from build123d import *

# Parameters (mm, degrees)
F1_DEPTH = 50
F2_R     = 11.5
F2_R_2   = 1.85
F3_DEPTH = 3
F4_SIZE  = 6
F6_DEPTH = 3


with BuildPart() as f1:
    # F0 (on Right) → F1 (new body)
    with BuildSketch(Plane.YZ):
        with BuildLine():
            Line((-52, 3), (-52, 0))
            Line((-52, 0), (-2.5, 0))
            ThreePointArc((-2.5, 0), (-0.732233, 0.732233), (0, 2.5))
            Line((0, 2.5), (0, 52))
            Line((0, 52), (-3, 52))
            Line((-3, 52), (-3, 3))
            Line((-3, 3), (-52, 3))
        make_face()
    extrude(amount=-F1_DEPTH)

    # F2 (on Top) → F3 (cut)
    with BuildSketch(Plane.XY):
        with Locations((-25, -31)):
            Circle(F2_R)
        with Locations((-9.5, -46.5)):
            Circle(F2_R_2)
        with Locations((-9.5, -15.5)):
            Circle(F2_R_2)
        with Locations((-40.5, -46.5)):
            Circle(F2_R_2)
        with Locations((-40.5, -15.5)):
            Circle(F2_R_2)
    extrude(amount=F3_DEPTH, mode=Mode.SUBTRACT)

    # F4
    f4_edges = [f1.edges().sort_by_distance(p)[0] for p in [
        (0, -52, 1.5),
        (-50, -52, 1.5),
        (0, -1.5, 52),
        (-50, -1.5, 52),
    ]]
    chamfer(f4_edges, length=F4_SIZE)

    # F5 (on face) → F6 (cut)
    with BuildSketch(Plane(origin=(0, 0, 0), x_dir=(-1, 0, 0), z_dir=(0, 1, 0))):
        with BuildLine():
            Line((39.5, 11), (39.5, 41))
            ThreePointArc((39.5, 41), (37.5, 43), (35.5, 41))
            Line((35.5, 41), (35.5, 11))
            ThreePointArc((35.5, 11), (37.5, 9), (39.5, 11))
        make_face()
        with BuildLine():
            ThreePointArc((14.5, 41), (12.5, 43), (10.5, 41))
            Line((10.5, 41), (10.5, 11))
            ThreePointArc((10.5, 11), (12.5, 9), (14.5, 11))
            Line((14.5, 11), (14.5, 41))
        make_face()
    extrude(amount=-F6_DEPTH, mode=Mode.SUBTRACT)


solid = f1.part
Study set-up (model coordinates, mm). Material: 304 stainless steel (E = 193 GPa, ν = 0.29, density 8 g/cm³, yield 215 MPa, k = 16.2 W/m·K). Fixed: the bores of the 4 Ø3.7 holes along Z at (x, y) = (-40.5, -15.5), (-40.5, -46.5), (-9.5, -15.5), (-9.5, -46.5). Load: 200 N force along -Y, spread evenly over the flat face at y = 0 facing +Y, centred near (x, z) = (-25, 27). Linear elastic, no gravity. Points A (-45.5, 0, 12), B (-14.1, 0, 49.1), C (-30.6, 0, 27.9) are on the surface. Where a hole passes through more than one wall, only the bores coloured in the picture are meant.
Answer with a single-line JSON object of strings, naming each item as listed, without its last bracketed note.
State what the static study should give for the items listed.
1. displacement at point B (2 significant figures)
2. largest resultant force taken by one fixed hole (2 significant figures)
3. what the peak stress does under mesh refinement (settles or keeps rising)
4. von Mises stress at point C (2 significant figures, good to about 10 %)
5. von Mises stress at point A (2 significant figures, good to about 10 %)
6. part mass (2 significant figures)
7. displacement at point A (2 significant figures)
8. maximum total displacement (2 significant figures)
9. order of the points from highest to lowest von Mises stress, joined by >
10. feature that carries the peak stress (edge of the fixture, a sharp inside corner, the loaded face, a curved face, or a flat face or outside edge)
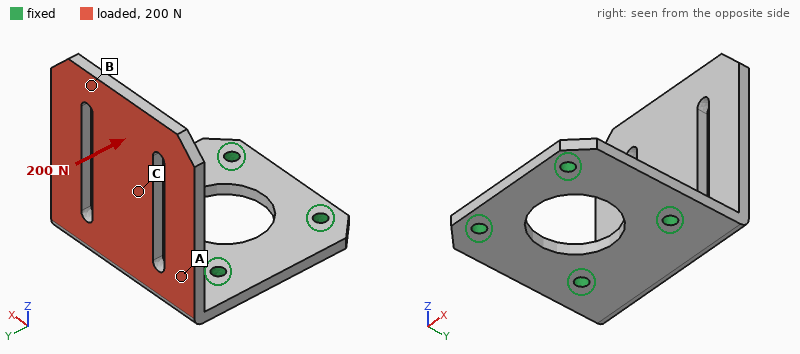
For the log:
{"displacement at point B": "0.30 mm", "largest resultant force taken by one fixed hole": "100 N", "what the peak stress does under mesh refinement": "keeps rising", "von Mises stress at point C": "19 MPa", "von Mises stress at point A": "49 MPa", "part mass": "100 g", "displacement at point A": "0.055 mm", "maximum total displacement": "0.32 mm", "order of the points from highest to lowest von Mises stress, joined by >": "A > C > B", "feature that carries the peak stress": "edge of the fixture"}
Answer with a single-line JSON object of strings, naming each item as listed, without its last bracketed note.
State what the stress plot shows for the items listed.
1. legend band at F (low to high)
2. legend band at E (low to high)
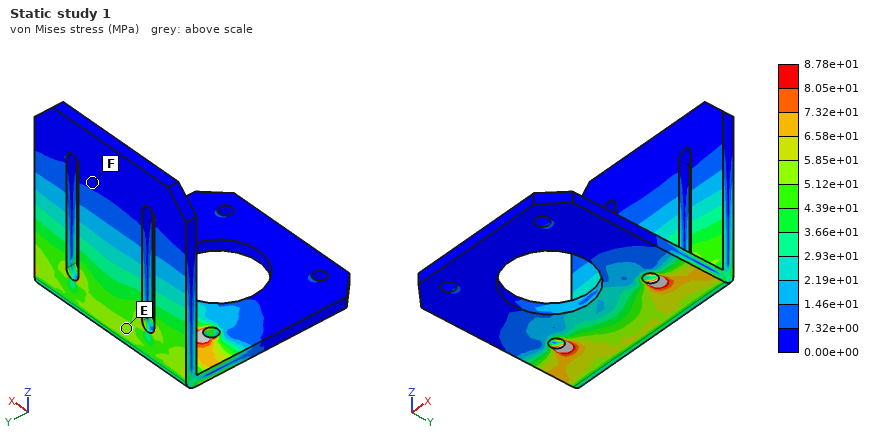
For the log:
{"legend band at F": "0.00e+00 to 7.32e+00 MPa", "legend band at E": "5.12e+01 to 5.85e+01 MPa"}
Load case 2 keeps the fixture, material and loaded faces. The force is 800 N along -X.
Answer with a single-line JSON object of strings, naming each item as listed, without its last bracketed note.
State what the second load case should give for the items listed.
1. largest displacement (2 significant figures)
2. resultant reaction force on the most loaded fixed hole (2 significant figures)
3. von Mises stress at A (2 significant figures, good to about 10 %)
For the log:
{"largest displacement": "0.12 mm", "resultant reaction force on the most loaded fixed hole": "790 N", "von Mises stress at A": "24 MPa"}
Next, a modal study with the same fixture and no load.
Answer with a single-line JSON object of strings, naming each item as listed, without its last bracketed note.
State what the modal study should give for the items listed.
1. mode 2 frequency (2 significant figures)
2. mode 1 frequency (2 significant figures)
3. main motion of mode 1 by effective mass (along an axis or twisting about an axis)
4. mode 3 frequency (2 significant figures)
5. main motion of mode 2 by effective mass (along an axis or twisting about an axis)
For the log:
{"mode 2 frequency": "1800 Hz", "mode 1 frequency": "670 Hz", "main motion of mode 1 by effective mass": "along Y", "mode 3 frequency": "2500 Hz", "main motion of mode 2 by effective mass": "along X"}
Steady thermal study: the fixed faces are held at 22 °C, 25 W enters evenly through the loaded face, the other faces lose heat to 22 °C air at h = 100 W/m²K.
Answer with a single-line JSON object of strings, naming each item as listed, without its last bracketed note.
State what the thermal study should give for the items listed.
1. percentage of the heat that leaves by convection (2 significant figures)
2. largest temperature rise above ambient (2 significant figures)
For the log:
{"percentage of the heat that leaves by convection": "87 %", "largest temperature rise above ambient": "77 K"}
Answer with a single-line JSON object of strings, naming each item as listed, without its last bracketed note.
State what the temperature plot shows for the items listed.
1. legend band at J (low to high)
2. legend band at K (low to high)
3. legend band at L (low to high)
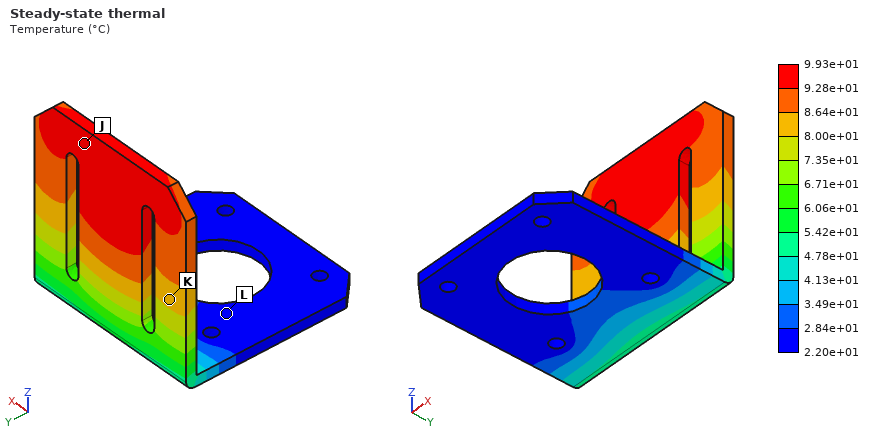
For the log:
{"legend band at J": "9.28e+01 to 9.93e+01 °C", "legend band at K": "8.00e+01 to 8.64e+01 °C", "legend band at L": "2.20e+01 to 2.84e+01 °C"}
